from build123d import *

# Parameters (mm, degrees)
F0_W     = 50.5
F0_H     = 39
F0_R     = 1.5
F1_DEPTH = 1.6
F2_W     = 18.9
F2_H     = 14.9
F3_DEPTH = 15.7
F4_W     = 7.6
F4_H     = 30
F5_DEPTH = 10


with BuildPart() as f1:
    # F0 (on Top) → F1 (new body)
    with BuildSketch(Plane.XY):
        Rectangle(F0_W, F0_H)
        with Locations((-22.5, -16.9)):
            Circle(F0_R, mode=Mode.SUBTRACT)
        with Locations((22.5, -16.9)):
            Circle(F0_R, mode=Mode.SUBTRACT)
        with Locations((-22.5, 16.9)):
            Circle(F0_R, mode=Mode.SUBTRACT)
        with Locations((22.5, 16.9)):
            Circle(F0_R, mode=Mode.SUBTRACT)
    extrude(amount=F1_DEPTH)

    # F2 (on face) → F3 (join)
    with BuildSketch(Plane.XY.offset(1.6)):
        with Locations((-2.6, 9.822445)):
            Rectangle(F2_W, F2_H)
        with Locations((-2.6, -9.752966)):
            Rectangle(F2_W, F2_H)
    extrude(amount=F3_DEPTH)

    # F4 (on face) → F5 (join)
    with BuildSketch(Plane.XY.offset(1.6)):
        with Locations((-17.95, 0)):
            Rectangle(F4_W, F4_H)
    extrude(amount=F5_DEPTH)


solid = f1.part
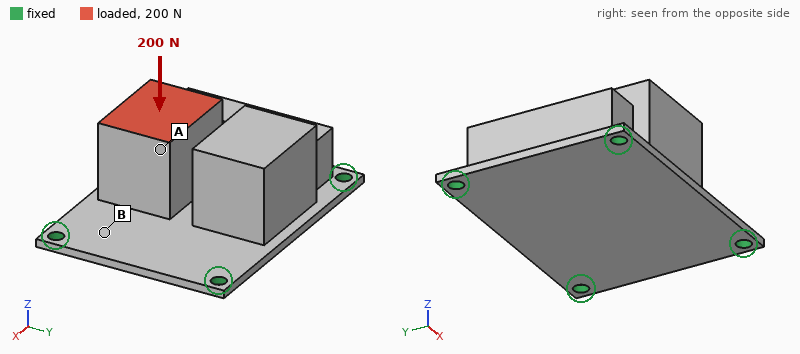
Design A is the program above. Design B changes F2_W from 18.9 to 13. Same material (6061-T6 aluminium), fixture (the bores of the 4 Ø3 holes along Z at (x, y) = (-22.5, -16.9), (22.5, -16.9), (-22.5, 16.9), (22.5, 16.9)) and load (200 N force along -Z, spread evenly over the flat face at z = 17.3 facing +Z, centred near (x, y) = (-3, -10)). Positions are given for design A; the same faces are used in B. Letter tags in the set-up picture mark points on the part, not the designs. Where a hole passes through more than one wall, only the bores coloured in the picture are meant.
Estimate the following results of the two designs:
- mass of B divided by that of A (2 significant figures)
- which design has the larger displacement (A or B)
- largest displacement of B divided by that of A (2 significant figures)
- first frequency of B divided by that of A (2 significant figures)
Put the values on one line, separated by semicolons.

0.81; B; 1.5; 0.95
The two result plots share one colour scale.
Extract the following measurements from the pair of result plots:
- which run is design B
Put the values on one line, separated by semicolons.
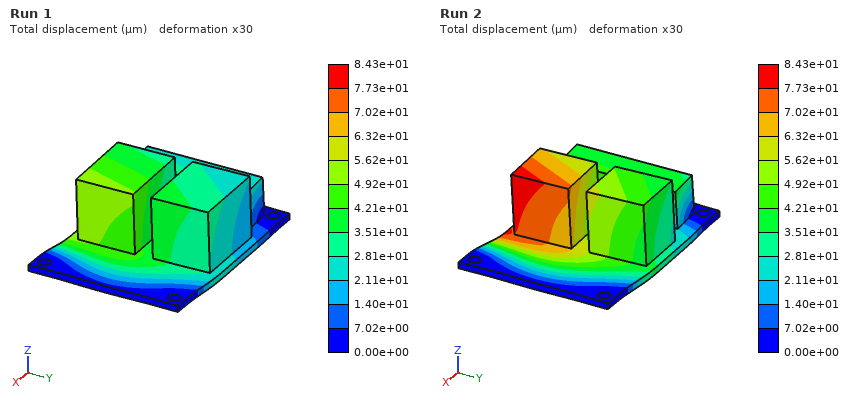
Run 2
